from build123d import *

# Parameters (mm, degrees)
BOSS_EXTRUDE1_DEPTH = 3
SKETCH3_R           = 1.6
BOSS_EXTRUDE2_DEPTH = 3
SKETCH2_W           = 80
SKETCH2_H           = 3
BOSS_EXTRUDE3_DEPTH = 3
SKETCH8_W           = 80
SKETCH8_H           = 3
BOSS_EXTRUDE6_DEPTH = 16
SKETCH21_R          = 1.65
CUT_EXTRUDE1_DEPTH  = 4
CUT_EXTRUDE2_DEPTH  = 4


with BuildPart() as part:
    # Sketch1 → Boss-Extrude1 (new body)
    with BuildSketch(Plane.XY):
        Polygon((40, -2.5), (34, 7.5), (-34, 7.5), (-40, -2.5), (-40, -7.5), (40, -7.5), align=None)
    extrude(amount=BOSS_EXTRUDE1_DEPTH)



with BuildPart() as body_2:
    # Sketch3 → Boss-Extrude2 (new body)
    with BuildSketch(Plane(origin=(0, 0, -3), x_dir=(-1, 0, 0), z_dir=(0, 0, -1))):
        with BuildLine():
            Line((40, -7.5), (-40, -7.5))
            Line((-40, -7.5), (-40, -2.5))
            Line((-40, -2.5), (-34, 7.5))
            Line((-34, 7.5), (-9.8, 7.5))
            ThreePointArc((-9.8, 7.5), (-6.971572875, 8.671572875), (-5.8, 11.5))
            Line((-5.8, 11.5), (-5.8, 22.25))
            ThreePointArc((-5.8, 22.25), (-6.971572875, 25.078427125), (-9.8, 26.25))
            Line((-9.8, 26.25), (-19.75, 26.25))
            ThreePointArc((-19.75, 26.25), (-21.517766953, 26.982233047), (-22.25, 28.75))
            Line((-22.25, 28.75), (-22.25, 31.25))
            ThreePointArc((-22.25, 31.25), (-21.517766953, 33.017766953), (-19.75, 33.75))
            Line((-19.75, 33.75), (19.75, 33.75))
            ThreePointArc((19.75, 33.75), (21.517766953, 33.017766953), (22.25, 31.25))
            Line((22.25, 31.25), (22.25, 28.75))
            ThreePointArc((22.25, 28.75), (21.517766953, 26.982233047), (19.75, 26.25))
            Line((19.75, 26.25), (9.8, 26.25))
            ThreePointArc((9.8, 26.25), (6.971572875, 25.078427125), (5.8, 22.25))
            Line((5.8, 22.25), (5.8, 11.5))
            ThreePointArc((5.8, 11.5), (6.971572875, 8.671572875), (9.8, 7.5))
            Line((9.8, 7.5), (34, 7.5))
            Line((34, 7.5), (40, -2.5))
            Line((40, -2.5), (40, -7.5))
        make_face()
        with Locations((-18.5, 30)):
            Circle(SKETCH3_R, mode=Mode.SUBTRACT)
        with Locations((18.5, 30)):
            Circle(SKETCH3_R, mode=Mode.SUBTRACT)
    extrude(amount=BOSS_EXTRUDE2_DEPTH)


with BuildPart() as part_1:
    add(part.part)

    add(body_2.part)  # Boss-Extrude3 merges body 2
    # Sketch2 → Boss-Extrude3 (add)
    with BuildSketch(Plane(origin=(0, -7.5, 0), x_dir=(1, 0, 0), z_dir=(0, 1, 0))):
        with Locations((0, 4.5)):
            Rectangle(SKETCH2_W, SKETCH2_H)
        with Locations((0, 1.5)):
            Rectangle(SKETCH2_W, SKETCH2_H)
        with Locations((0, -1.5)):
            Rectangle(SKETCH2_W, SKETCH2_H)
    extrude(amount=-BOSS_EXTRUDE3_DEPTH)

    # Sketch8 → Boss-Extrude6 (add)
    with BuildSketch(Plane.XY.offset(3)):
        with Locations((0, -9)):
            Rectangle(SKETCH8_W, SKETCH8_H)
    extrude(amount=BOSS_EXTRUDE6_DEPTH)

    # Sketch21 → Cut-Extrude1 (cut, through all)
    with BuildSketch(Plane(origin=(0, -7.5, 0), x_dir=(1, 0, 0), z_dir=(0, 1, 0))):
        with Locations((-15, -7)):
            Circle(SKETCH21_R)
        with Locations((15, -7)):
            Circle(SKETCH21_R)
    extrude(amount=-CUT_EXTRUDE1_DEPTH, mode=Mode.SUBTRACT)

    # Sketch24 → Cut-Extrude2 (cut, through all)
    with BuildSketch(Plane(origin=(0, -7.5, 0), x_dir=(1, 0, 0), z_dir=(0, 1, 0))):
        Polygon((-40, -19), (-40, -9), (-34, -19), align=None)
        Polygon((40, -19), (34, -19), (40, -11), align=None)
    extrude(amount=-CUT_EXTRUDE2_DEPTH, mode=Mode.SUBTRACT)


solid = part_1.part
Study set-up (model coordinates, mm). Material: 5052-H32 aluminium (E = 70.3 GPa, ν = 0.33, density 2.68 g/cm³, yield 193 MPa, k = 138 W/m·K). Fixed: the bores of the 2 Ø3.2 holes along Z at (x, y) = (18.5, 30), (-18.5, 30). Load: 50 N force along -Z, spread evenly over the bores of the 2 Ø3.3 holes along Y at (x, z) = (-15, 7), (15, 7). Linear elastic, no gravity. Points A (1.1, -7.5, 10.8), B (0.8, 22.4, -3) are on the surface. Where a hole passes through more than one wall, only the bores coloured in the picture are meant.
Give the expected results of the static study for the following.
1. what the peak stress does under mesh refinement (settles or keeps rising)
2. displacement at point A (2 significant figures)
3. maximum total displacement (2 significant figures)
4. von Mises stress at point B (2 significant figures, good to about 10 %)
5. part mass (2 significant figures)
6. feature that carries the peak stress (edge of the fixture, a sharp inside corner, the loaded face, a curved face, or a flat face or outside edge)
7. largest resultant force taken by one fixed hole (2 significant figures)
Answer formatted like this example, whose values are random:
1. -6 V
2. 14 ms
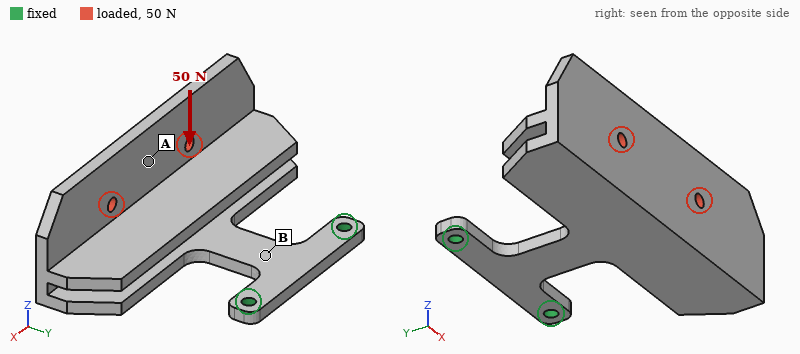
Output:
1. keeps rising
2. 0.83 mm
3. 1.00 mm
4. 87 MPa
5. 38 g
6. edge of the fixture
7. 25 N
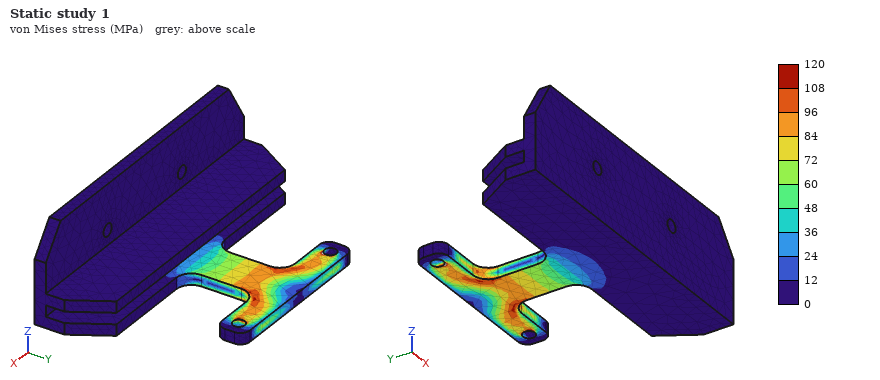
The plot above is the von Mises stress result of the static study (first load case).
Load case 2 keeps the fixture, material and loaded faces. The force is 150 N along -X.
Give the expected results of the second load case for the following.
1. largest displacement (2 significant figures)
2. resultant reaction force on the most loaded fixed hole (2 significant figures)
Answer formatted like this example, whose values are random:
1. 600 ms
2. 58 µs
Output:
1. 0.84 mm
2. 230 N
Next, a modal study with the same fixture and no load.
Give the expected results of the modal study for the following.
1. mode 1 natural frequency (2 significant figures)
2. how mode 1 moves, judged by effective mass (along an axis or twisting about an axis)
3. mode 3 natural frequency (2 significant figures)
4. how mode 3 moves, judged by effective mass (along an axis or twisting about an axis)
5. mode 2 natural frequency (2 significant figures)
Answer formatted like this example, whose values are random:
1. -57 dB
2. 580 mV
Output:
1. 240 Hz
2. along Z
3. 880 Hz
4. along X
5. 350 Hz
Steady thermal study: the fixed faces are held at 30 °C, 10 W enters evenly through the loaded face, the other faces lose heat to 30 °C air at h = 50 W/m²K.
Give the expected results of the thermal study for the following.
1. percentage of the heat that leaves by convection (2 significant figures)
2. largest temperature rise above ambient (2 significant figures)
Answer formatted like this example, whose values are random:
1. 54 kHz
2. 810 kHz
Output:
1. 80 %
2. 22 K
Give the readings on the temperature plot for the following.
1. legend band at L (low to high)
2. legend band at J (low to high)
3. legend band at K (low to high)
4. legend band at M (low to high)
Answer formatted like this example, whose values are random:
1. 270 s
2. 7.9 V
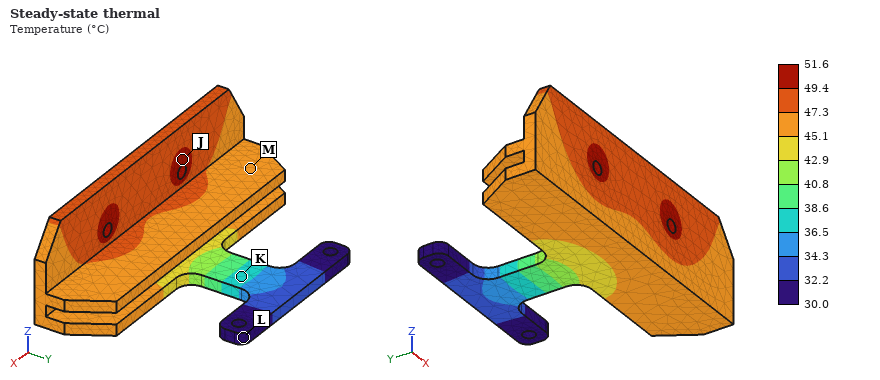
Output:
1. 30.0 to 32.2 °C
2. 49.4 to 51.6 °C
3. 36.5 to 38.6 °C
4. 45.1 to 47.3 °C
